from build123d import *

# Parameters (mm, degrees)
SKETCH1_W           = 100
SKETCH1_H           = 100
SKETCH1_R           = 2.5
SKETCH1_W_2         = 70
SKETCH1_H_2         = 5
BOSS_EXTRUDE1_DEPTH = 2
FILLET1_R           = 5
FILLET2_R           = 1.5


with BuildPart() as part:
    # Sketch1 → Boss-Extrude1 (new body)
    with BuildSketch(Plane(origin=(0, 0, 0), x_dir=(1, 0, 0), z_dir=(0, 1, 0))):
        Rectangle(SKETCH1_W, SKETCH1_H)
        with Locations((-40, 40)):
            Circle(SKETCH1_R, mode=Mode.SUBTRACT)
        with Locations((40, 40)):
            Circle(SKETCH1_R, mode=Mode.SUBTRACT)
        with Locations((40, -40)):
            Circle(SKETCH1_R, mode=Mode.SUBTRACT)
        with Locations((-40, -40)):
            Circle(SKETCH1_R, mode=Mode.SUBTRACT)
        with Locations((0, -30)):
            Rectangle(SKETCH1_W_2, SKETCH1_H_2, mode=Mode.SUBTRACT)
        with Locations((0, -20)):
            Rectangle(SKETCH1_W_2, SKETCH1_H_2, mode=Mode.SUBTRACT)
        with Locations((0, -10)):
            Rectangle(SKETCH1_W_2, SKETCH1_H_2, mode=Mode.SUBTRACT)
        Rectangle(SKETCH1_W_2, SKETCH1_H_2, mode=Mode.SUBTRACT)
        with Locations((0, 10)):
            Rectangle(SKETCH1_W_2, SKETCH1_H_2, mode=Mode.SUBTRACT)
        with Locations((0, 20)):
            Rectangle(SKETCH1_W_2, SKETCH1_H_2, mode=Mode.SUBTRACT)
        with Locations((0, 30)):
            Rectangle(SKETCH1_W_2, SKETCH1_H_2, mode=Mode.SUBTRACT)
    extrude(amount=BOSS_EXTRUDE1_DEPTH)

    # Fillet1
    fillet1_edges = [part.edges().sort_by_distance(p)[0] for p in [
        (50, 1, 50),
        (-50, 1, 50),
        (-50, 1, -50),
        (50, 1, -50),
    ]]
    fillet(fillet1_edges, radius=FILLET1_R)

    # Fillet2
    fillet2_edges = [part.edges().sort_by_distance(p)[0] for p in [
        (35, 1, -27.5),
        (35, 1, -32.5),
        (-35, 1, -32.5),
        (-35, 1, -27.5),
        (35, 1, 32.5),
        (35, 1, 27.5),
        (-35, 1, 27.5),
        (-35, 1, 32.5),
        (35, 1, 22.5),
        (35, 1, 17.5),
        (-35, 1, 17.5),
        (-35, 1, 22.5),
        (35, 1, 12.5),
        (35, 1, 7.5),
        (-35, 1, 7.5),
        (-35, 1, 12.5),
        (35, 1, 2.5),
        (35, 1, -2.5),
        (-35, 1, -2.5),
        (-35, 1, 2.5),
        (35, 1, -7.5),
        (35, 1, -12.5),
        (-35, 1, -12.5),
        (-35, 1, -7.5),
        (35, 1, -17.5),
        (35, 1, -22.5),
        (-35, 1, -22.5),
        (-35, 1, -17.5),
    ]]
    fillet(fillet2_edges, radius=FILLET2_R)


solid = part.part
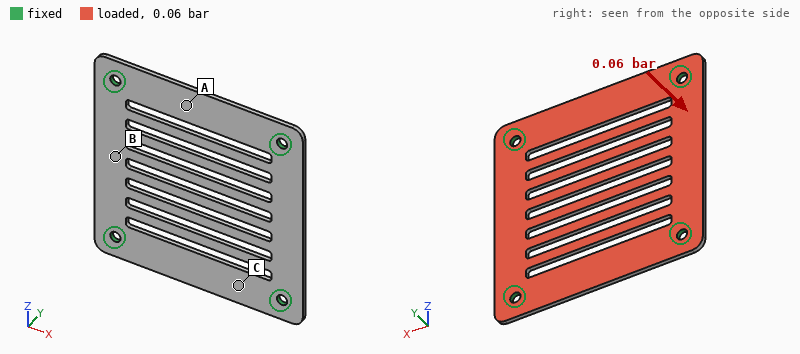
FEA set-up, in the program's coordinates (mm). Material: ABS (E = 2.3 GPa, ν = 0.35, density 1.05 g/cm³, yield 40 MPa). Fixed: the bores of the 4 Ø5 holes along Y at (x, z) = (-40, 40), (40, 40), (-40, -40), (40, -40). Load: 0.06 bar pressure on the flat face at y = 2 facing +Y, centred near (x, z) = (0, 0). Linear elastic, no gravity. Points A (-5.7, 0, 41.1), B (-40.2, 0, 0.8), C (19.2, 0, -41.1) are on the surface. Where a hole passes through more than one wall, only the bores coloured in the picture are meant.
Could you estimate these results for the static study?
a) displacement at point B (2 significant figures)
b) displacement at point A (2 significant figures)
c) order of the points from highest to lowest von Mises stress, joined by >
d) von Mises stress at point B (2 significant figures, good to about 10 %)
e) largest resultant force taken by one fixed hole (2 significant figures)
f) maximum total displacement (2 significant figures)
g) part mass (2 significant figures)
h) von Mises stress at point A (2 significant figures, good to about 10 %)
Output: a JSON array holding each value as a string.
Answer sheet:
["0.71 mm", "0.31 mm", "B > A > C", "4.7 MPa", "11 N", "1.6 mm", "16 g", "1.8 MPa"]
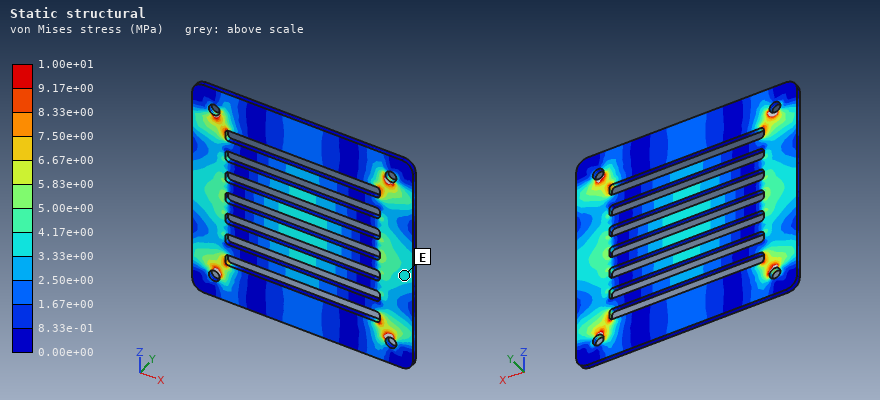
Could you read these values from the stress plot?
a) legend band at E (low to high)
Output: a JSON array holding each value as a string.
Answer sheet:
["3.33e+00 to 4.17e+00 MPa"]
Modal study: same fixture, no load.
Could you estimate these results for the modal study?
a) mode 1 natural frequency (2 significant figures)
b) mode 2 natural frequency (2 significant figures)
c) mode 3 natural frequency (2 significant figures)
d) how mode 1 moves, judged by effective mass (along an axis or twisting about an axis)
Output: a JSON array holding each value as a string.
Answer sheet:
["270 Hz", "420 Hz", "470 Hz", "along Y"]
